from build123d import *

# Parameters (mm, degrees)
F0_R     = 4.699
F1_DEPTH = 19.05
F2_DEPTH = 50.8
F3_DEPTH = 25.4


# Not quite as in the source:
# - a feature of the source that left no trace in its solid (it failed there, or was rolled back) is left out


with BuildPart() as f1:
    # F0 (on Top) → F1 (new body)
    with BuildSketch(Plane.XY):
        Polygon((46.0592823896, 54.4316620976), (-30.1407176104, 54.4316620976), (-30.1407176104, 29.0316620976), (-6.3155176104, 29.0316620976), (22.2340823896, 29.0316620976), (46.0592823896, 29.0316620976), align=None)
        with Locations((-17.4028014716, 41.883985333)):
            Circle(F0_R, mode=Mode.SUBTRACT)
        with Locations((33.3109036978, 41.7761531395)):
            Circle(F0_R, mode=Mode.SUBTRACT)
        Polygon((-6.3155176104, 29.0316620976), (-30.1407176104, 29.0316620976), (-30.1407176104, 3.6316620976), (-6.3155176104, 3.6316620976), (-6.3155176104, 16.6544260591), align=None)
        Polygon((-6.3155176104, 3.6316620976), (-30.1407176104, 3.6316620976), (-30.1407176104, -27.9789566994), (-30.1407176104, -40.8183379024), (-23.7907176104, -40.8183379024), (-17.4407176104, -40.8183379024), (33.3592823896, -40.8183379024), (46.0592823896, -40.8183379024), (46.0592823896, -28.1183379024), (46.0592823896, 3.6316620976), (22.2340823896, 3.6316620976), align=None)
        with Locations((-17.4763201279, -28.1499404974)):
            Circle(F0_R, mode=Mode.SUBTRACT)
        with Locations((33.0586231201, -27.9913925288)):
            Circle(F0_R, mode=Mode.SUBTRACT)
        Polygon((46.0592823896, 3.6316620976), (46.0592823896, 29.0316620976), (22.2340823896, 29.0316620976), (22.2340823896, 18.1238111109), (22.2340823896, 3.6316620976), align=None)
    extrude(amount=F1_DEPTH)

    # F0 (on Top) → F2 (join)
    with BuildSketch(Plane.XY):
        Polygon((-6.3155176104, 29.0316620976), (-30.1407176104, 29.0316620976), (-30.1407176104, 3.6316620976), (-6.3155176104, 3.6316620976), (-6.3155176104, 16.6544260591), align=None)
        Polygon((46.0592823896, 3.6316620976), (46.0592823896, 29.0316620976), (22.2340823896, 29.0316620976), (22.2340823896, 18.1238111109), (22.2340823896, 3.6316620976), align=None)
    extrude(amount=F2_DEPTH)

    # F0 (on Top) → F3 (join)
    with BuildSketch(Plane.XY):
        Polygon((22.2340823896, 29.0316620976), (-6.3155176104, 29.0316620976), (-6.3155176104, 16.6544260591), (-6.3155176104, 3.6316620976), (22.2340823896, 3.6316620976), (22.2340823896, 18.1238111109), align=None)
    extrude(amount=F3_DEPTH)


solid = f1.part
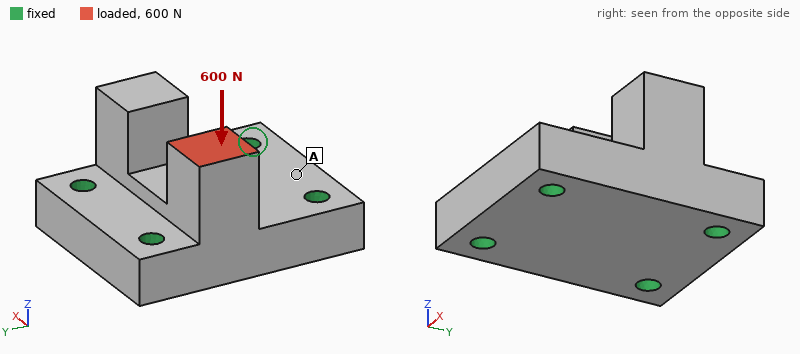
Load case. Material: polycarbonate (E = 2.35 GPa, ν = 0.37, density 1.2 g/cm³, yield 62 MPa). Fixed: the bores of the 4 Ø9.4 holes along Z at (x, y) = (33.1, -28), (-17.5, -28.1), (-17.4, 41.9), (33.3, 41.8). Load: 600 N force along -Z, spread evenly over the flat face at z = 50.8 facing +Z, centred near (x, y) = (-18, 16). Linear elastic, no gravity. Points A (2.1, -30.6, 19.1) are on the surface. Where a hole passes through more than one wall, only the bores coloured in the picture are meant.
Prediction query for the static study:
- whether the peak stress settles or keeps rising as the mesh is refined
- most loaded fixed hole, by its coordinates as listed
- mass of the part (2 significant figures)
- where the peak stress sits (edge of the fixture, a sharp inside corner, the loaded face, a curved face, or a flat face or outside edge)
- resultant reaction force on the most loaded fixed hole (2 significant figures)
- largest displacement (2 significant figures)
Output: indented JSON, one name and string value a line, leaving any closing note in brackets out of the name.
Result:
{
  "whether the peak stress settles or keeps rising as the mesh is refined": "keeps rising",
  "most loaded fixed hole, by its coordinates as listed": "(-17.4, 41.9)",
  "mass of the part": "210 g",
  "where the peak stress sits": "edge of the fixture",
  "resultant reaction force on the most loaded fixed hole": "390 N",
  "largest displacement": "62 µm"
}
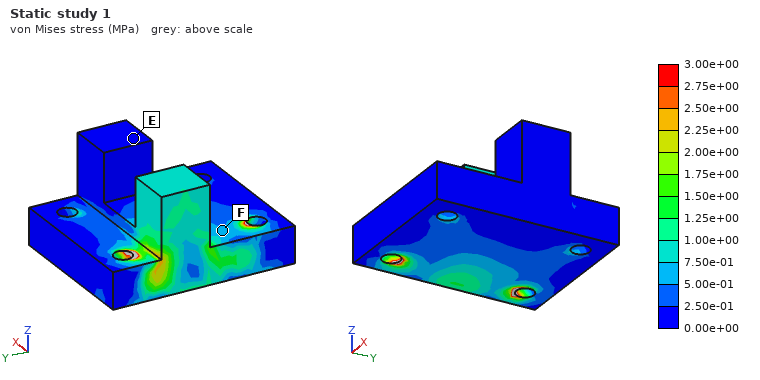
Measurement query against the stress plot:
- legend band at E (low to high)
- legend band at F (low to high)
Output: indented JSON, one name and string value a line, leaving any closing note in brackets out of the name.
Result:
{
  "legend band at E": "0.00e+00 to 2.50e-01 MPa",
  "legend band at F": "5.00e-01 to 7.50e-01 MPa"
}
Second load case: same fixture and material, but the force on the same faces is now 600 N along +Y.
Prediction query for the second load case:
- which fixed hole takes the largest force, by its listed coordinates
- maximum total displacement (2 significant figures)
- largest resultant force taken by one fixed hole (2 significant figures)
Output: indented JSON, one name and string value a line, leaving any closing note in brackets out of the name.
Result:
{
  "which fixed hole takes the largest force, by its listed coordinates": "(-17.4, 41.9)",
  "maximum total displacement": "0.24 mm",
  "largest resultant force taken by one fixed hole": "480 N"
}
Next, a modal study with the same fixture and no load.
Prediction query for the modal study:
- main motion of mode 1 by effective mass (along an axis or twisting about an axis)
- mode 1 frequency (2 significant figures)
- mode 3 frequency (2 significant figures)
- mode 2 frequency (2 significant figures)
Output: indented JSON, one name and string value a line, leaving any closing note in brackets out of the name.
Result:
{
  "main motion of mode 1 by effective mass": "along X",
  "mode 1 frequency": "2300 Hz",
  "mode 3 frequency": "2800 Hz",
  "mode 2 frequency": "2600 Hz"
}
